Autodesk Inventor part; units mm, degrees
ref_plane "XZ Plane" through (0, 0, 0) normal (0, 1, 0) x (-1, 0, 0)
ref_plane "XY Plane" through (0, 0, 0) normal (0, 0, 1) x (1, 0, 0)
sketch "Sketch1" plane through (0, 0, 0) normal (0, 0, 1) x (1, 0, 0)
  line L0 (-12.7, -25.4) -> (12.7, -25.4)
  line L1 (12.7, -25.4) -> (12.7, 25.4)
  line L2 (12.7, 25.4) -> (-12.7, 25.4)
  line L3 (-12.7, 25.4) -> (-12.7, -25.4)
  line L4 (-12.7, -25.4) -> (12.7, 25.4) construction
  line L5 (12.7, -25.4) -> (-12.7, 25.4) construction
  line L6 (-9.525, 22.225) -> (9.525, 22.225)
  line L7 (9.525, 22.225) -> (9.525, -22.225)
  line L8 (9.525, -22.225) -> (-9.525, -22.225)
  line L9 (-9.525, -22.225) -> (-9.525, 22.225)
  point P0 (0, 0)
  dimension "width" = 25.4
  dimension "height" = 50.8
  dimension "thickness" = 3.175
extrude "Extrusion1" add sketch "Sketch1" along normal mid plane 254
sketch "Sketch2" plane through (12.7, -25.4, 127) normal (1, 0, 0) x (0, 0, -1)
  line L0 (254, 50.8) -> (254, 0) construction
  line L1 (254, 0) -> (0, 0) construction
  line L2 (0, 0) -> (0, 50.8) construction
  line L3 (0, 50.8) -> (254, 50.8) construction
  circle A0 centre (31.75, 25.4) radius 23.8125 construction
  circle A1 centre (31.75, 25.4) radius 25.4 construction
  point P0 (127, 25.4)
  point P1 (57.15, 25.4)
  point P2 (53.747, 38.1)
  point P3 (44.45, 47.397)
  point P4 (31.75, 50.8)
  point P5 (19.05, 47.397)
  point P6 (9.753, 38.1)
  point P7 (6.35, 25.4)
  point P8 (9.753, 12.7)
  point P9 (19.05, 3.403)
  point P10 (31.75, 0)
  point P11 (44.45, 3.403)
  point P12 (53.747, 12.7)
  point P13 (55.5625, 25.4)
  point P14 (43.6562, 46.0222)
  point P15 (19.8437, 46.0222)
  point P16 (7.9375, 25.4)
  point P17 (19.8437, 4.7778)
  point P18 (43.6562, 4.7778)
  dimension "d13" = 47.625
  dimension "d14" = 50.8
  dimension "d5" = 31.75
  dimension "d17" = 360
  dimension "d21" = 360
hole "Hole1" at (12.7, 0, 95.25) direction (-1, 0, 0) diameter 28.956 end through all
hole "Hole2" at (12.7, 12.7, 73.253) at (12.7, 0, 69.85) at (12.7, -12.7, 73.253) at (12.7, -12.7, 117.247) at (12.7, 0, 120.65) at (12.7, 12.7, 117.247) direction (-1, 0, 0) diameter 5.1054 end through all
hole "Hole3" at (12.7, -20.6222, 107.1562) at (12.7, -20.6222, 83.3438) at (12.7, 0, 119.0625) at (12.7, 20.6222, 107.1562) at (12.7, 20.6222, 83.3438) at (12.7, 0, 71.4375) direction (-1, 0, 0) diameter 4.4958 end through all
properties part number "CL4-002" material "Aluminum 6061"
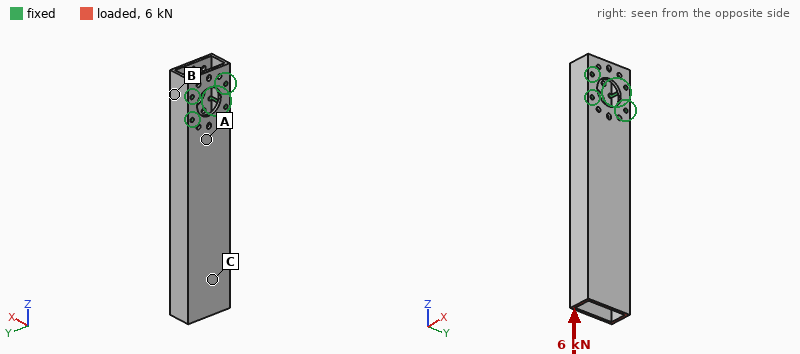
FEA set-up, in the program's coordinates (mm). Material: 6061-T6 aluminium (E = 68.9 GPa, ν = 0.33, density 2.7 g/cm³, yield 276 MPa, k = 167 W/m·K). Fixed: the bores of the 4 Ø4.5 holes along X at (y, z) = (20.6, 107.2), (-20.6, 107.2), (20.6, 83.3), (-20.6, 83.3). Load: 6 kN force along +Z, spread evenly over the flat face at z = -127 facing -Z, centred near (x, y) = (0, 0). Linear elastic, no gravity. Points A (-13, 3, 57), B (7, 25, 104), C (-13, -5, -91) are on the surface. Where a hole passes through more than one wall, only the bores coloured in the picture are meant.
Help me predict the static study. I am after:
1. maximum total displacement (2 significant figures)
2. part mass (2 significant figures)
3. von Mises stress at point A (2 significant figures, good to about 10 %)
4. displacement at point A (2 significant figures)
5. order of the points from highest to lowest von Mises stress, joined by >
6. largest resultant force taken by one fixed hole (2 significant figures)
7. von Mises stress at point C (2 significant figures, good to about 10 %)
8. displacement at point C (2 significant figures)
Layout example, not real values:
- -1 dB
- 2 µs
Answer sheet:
- 43 µm
- 290 g
- 9.4 MPa
- 8.1 µm
- C > A > B
- 2.8 kN
- 14 MPa
- 36 µm
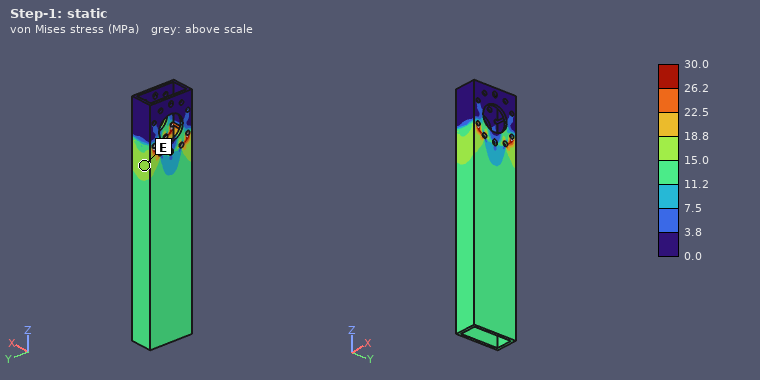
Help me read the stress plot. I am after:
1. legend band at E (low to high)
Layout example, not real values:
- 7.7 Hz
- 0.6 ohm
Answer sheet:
- 15.0 to 18.8 MPa
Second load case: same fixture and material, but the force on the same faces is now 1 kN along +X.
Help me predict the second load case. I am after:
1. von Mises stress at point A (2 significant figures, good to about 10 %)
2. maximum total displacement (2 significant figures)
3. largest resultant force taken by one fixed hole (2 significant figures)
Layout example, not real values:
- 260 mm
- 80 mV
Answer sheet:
- 39 MPa
- 1.3 mm
- 630 N
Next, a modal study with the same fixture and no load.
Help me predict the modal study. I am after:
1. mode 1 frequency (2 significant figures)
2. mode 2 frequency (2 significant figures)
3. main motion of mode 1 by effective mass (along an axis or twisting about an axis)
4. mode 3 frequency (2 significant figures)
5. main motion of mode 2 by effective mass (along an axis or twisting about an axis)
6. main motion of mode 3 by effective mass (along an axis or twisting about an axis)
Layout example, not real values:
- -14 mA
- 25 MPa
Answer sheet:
- 550 Hz
- 1000 Hz
- along X
- 2500 Hz
- along Y
- twisting about Z
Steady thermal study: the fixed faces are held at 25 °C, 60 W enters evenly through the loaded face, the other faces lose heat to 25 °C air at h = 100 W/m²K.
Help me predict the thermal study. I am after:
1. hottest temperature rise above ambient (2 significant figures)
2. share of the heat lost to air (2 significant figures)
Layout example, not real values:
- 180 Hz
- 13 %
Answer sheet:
- 42 K
- 97 %
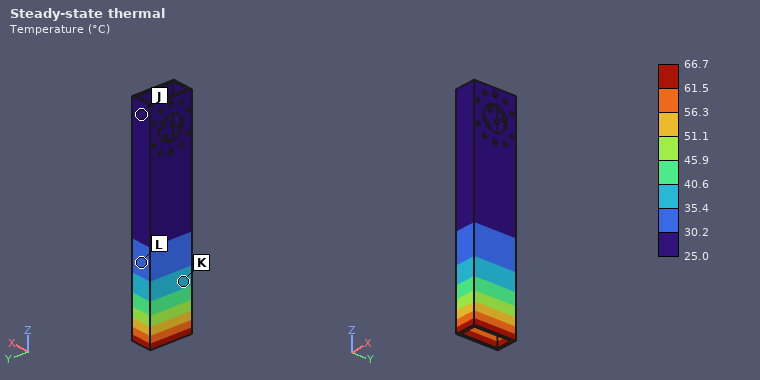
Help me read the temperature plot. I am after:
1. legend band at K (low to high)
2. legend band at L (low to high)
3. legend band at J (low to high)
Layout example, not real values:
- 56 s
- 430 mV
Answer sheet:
- 35.4 to 40.6 °C
- 30.2 to 35.4 °C
- 25.0 to 30.2 °C
